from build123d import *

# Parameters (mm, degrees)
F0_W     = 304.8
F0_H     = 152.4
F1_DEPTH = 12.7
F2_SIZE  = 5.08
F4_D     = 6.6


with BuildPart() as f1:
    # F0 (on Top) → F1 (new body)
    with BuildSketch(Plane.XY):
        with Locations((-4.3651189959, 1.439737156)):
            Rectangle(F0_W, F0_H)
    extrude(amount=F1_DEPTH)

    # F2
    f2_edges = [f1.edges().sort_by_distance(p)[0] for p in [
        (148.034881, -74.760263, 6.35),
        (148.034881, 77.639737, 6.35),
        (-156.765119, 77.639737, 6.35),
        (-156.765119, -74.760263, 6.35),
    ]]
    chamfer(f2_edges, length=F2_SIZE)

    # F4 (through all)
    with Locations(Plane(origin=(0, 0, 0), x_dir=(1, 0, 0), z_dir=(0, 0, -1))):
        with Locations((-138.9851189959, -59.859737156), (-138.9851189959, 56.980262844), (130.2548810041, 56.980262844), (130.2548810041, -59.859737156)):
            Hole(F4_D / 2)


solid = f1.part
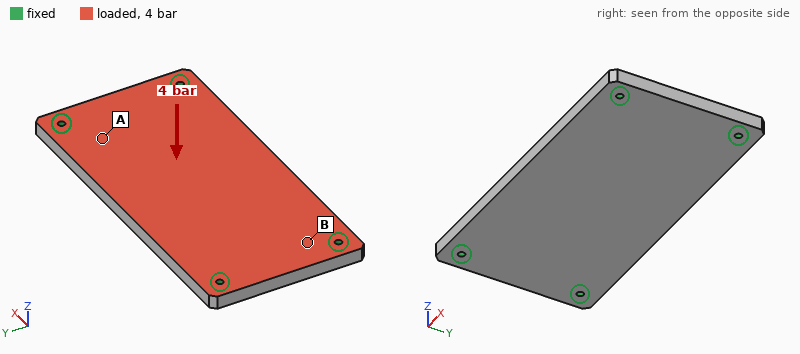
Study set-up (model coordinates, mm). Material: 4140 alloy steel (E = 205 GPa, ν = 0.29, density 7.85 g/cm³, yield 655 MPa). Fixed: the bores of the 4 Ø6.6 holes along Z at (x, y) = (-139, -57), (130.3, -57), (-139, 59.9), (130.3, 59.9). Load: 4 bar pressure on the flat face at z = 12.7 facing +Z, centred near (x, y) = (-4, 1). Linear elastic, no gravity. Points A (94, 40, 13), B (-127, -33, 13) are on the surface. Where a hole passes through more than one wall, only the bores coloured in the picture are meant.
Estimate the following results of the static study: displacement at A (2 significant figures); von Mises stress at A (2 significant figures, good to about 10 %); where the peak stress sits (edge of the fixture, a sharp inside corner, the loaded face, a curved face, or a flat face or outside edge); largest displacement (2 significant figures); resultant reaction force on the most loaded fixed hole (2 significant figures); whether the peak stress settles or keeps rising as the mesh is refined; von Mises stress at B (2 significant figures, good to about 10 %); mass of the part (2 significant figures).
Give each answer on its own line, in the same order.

0.070 mm
20 MPa
edge of the fixture
0.23 mm
4.6 kN
keeps rising
42 MPa
4.6 kg
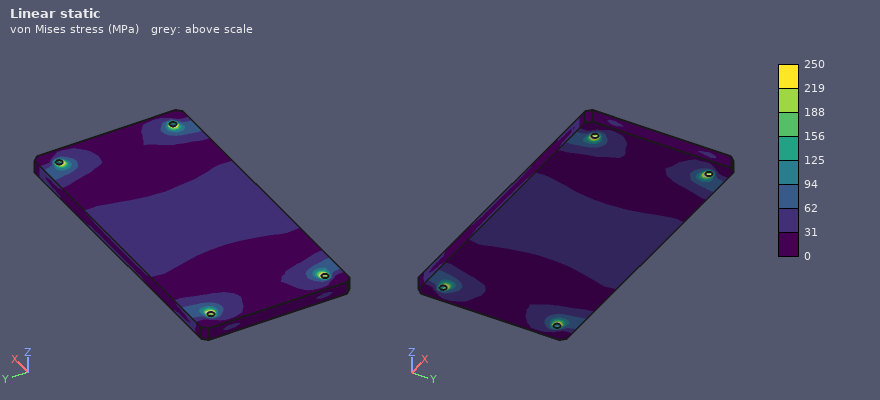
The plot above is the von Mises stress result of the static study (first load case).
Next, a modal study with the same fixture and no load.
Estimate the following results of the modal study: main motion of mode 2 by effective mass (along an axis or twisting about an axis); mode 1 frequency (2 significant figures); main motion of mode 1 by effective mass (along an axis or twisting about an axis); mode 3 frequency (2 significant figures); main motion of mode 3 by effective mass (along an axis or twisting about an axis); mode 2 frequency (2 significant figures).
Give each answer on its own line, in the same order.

twisting about X
770 Hz
along Z
2100 Hz
twisting about Y
1300 Hz
